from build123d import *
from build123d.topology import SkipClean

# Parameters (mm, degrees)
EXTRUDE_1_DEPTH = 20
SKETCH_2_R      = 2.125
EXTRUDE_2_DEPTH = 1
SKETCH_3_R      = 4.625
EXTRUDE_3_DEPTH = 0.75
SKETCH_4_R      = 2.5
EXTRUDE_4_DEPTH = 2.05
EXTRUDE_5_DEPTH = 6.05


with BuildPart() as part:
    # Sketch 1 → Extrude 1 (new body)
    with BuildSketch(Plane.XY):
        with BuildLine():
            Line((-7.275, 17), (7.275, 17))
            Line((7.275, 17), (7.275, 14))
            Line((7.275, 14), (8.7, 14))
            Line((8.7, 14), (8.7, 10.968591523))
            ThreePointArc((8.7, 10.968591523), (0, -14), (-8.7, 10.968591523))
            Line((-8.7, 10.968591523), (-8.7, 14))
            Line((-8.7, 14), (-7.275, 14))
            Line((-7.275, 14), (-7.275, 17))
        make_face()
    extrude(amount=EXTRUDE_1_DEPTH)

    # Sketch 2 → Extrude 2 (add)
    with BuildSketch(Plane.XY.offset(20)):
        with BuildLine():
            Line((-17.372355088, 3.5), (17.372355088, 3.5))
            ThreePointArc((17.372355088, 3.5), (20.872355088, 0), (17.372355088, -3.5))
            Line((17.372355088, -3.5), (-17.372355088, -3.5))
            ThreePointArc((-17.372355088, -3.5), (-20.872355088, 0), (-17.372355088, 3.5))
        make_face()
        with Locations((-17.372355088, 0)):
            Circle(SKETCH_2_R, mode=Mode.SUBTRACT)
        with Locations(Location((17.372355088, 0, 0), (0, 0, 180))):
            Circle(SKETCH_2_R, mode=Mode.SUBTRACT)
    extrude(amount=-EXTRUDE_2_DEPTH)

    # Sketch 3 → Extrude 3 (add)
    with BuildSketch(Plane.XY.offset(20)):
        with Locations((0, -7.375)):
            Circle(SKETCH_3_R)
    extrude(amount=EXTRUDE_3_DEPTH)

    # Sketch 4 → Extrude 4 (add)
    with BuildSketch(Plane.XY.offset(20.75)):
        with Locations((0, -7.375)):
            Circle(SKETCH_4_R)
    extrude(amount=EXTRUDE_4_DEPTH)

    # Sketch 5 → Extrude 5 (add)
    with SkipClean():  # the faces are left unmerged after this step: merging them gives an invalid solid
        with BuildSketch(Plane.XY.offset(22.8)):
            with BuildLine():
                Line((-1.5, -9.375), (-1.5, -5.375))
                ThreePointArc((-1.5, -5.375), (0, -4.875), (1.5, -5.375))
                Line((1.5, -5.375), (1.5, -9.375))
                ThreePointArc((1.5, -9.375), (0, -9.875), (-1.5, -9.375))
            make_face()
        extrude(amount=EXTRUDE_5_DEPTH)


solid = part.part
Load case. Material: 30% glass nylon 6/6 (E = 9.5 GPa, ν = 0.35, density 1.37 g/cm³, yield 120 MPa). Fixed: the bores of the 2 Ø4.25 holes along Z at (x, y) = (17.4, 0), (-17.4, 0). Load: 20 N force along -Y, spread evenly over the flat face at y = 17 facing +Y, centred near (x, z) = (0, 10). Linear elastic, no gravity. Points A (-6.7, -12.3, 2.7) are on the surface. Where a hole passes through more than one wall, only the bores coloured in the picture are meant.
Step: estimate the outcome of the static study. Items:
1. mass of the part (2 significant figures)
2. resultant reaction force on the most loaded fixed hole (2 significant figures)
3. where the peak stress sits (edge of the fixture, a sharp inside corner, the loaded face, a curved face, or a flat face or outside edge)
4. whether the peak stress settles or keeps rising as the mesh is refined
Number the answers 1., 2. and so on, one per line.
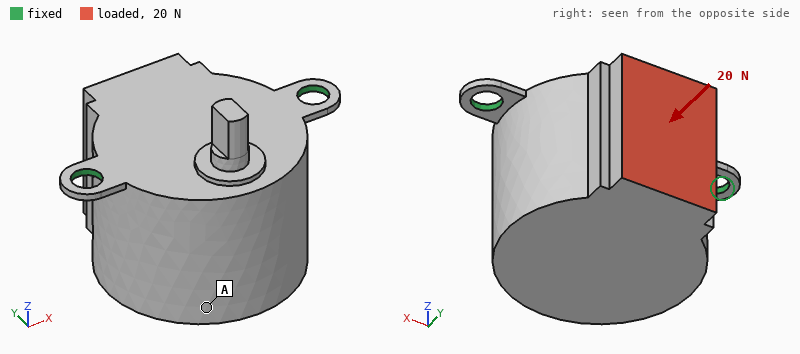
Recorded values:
1. 19 g
2. 10 N
3. edge of the fixture
4. keeps rising
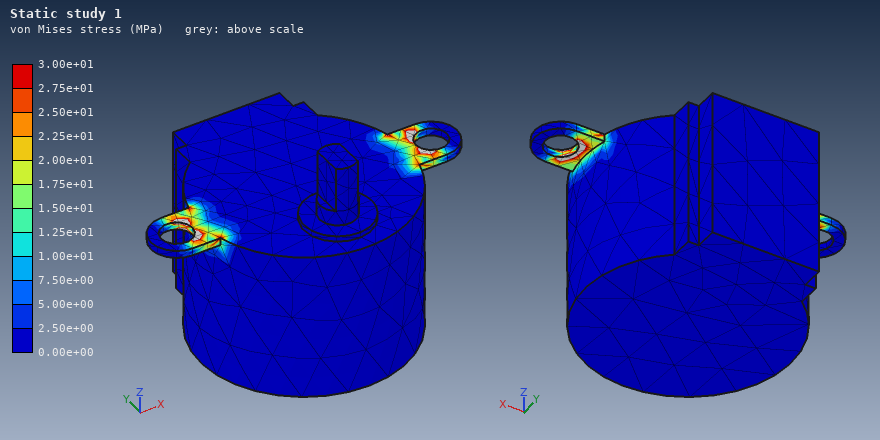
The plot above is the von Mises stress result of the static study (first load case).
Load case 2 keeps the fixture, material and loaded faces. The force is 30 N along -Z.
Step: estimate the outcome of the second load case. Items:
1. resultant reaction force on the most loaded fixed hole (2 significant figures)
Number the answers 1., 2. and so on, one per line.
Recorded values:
1. 18 N
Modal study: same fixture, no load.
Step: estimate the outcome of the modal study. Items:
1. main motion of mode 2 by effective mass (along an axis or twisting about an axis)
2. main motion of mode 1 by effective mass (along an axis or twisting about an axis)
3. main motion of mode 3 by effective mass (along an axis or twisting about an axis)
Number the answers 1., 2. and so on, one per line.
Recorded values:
1. along Z
2. along Y
3. along X
